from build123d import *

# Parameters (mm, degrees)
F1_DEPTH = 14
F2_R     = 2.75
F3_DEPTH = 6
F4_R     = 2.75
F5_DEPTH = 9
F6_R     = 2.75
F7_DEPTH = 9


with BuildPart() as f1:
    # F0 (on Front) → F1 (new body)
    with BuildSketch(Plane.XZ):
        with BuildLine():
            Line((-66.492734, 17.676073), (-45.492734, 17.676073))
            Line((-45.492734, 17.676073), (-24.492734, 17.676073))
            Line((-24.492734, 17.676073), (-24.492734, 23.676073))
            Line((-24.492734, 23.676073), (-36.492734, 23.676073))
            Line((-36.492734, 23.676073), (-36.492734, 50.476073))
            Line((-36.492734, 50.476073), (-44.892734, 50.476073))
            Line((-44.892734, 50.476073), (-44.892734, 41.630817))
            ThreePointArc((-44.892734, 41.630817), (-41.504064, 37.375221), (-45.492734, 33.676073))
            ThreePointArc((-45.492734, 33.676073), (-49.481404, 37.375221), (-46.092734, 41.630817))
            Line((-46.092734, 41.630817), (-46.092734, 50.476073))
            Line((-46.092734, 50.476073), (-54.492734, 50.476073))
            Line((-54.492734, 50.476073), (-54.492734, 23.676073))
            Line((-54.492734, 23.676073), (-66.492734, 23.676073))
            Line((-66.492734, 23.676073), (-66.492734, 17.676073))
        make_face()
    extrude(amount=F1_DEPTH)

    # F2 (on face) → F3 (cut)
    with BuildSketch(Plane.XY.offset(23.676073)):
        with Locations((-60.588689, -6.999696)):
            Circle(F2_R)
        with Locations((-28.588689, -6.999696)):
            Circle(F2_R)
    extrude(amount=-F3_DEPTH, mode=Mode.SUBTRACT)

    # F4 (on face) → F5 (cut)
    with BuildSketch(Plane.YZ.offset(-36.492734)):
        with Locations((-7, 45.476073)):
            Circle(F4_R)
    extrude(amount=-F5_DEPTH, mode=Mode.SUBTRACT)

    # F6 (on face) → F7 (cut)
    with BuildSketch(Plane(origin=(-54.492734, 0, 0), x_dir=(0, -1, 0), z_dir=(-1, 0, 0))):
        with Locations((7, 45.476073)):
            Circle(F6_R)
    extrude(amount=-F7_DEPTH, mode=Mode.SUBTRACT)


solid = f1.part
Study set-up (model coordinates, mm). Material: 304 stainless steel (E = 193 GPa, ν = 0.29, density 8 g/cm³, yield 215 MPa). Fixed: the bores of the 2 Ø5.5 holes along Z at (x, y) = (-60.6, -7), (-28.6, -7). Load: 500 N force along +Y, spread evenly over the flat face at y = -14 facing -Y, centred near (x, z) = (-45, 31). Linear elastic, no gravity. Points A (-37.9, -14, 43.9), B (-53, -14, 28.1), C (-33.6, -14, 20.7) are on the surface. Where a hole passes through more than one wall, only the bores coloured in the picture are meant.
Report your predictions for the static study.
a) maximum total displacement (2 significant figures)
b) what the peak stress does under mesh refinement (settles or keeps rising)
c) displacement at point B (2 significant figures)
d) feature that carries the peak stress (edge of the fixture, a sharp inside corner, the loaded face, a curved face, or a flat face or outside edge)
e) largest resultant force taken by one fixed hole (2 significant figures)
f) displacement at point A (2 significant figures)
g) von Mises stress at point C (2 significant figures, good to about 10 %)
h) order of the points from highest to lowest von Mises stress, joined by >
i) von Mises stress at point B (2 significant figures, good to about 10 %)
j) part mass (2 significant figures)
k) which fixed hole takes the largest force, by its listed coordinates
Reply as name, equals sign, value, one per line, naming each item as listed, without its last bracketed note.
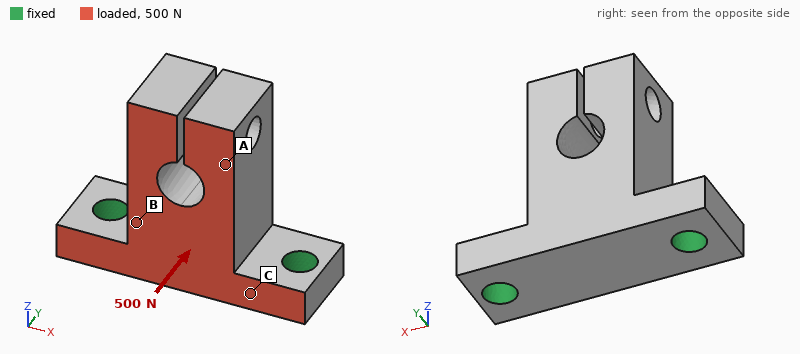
maximum total displacement = 11 µm
what the peak stress does under mesh refinement = keeps rising
displacement at point B = 3.3 µm
feature that carries the peak stress = edge of the fixture
largest resultant force taken by one fixed hole = 270 N
displacement at point A = 8.4 µm
von Mises stress at point C = 22 MPa
order of the points from highest to lowest von Mises stress, joined by > = C > B > A
von Mises stress at point B = 7.7 MPa
part mass = 70 g
which fixed hole takes the largest force, by its listed coordinates = (-60.6, -7)
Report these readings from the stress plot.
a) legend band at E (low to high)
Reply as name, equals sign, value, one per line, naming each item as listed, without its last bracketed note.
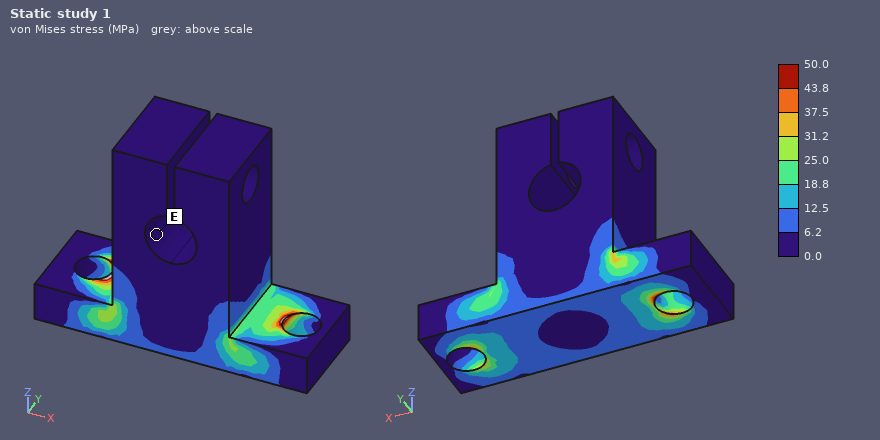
legend band at E = 0.0 to 6.2 MPa
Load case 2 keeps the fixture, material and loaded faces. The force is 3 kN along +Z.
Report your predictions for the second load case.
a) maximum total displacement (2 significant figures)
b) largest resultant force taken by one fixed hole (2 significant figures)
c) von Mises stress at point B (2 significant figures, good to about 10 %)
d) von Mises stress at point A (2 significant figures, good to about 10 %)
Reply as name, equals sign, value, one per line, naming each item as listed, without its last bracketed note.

maximum total displacement = 37 µm
largest resultant force taken by one fixed hole = 1.6 kN
von Mises stress at point B = 40 MPa
von Mises stress at point A = 16 MPa
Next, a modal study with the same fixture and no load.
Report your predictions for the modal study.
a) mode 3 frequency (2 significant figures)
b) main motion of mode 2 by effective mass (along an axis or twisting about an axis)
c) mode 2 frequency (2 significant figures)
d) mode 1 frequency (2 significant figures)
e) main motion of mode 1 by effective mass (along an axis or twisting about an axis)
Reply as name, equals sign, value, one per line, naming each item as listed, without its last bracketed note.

mode 3 frequency = 10 kHz
main motion of mode 2 by effective mass = along X
mode 2 frequency = 8200 Hz
mode 1 frequency = 5100 Hz
main motion of mode 1 by effective mass = along Y
